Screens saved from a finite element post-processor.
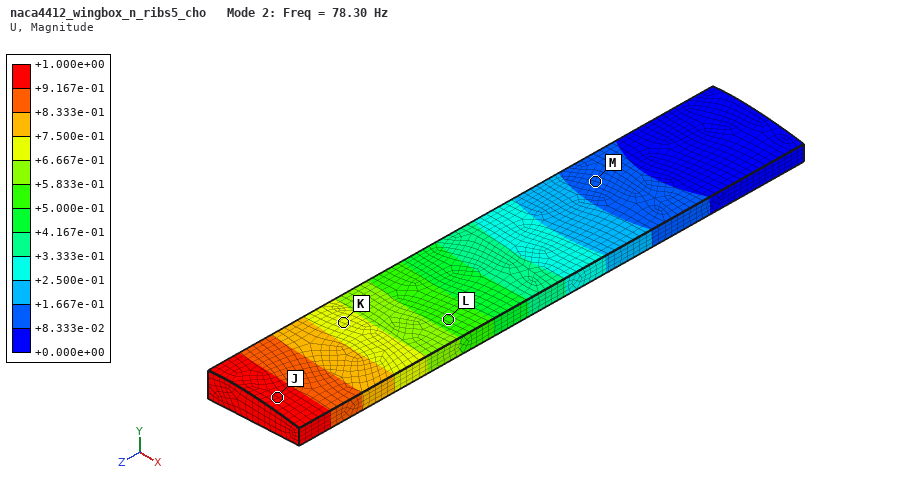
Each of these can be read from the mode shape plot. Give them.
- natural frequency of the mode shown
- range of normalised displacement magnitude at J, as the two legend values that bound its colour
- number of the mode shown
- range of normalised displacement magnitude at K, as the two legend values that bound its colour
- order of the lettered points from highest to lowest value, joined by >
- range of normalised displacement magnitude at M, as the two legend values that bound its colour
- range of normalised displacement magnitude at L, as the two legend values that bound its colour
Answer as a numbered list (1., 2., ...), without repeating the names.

1. 78.30 Hz
2. +9.167e-01 to +1.000e+00
3. 2
4. +6.667e-01 to +7.500e-01
5. J > K > L > M
6. +8.333e-02 to +1.667e-01
7. +5.000e-01 to +5.833e-01
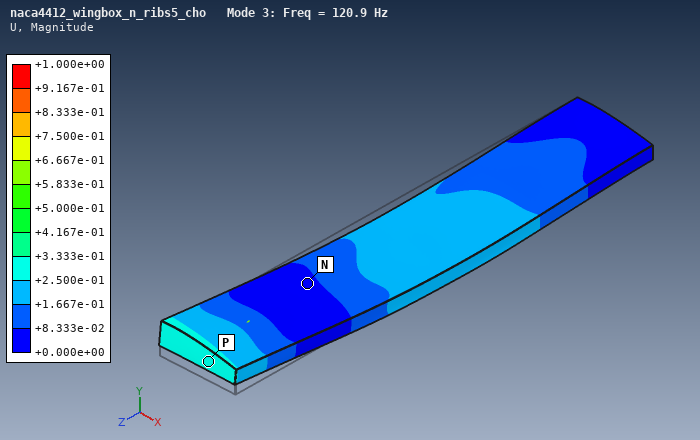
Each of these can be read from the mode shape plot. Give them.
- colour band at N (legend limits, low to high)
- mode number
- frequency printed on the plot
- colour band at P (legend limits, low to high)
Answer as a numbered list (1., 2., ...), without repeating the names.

1. +0.000e+00 to +8.333e-02
2. 3
3. 120.9 Hz
4. +2.500e-01 to +3.333e-01
